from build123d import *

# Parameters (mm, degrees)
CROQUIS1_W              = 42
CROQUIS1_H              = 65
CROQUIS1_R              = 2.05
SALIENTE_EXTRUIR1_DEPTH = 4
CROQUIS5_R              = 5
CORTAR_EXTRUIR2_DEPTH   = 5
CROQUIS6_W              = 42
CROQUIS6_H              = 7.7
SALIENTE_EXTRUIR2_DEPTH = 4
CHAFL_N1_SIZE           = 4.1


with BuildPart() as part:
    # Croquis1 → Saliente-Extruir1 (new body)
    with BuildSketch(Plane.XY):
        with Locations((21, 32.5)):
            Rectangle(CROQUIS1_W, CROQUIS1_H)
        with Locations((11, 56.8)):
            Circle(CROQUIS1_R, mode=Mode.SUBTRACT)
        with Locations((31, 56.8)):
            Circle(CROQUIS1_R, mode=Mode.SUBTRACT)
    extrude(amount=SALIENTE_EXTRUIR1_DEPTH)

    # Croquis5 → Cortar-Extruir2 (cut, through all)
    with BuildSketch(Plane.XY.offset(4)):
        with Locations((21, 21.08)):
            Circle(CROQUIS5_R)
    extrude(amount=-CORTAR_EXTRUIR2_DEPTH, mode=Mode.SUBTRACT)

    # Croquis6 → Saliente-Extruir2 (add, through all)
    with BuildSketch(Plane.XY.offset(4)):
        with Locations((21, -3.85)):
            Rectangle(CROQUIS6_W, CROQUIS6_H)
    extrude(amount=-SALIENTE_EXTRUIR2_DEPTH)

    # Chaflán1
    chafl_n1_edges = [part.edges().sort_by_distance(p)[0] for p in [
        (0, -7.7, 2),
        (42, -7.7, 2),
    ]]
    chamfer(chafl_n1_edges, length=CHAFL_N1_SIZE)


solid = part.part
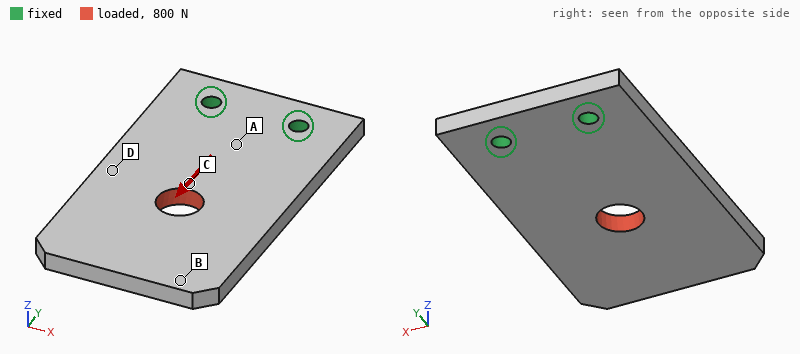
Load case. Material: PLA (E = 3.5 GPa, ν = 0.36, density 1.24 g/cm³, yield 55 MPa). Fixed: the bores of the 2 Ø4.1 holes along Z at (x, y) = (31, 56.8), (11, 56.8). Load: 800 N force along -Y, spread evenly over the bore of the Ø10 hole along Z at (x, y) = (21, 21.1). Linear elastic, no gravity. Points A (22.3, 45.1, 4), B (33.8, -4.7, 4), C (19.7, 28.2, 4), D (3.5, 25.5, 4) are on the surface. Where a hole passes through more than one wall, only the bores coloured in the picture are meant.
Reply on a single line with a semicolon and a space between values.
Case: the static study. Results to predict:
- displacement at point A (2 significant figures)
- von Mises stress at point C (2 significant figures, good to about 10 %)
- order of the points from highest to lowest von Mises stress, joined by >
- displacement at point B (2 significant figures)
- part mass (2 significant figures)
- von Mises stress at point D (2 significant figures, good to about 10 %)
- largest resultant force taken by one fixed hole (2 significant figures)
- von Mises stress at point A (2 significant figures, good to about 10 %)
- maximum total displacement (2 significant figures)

22 µm; 7.1 MPa; C > A > D > B; 59 µm; 15 g; 2.6 MPa; 400 N; 5.2 MPa; 80 µm
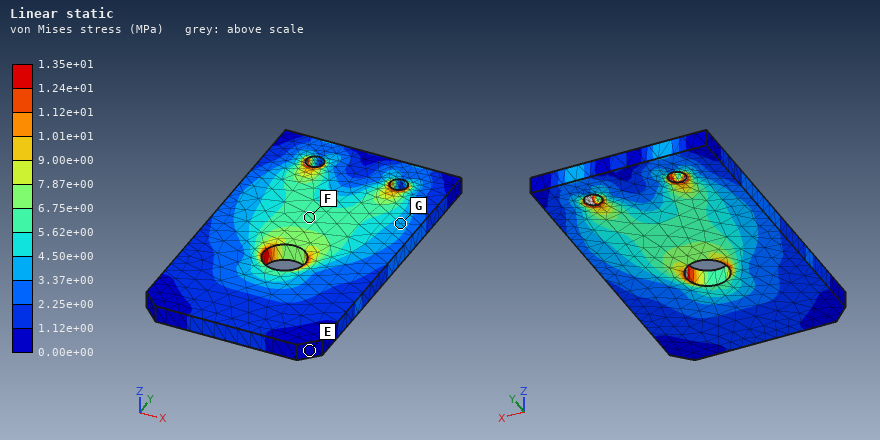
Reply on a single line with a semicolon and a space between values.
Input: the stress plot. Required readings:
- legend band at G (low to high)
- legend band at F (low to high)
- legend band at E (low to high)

3.37e+00 to 4.50e+00 MPa; 5.62e+00 to 6.75e+00 MPa; 0.00e+00 to 1.12e+00 MPa
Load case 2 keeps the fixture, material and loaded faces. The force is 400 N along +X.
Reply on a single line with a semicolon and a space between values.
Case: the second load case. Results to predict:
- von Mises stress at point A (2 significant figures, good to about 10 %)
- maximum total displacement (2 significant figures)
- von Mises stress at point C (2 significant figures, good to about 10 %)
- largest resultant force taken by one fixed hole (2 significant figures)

8.7 MPa; 0.38 mm; 8.5 MPa; 650 N
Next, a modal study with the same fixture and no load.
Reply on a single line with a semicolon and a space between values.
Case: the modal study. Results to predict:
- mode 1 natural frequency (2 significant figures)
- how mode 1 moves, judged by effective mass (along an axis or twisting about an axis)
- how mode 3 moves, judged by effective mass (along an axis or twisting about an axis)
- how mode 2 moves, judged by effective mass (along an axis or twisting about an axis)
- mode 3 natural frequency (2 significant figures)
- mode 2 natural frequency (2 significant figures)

270 Hz; along Z; along Z; twisting about Y; 1600 Hz; 850 Hz
